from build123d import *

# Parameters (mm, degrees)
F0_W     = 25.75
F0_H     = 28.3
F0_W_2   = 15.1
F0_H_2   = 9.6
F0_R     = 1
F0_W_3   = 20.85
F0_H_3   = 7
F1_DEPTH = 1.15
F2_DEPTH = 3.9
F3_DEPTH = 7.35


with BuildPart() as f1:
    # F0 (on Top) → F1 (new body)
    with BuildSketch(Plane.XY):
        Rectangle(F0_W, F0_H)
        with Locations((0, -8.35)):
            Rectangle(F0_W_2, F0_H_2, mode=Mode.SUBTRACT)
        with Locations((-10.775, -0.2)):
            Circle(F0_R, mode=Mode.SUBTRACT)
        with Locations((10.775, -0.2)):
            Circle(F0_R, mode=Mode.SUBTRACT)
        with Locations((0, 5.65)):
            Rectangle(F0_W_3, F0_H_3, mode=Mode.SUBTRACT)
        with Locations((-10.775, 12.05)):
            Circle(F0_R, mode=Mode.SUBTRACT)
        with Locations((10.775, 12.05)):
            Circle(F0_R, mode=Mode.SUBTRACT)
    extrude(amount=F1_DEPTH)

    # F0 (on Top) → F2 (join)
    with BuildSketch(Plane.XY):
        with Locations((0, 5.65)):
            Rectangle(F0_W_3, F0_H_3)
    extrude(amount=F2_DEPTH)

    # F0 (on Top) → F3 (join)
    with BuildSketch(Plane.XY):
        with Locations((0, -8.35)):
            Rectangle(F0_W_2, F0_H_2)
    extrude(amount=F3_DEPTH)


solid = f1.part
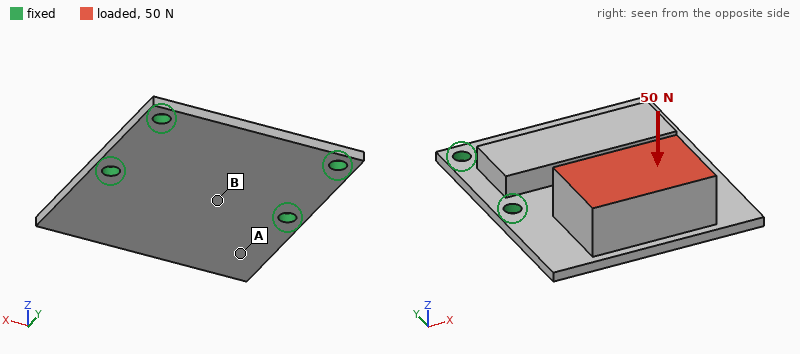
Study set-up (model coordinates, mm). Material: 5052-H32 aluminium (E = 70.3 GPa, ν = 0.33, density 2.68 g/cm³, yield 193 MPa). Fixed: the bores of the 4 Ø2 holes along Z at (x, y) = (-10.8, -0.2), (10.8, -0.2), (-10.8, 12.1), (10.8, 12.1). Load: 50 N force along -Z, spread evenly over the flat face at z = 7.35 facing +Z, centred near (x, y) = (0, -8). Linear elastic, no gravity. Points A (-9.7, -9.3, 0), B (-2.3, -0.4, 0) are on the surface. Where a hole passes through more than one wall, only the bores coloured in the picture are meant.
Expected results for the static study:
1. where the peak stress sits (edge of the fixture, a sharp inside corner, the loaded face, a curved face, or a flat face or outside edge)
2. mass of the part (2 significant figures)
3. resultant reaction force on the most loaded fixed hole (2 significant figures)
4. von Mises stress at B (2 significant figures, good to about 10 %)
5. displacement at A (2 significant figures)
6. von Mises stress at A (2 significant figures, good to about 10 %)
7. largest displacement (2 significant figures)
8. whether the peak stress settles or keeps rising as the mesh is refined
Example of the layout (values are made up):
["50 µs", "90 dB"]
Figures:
["edge of the fixture", "5.7 g", "32 N", "31 MPa", "44 µm", "11 MPa", "78 µm", "keeps rising"]
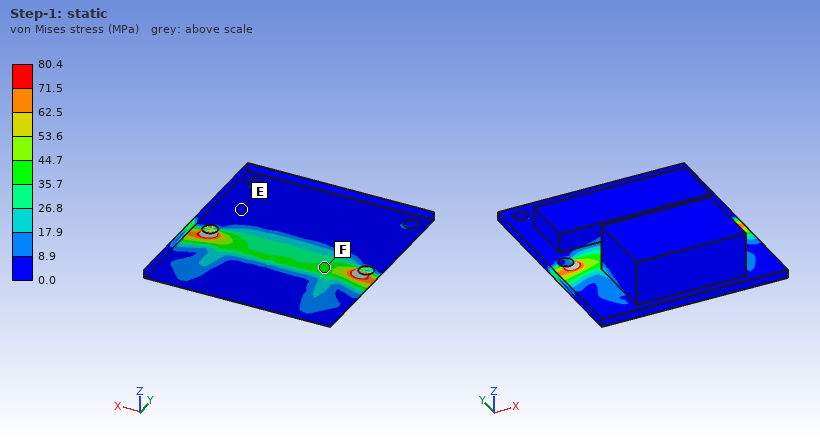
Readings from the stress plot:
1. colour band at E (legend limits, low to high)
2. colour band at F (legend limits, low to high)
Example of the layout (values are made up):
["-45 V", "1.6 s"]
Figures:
["0.0 to 8.9 MPa", "35.7 to 44.7 MPa"]
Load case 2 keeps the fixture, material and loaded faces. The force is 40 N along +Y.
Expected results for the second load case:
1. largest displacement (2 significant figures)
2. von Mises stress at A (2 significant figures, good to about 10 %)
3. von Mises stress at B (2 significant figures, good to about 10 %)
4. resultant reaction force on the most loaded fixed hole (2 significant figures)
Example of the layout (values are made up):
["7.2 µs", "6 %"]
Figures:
["64 µm", "6.9 MPa", "26 MPa", "14 N"]
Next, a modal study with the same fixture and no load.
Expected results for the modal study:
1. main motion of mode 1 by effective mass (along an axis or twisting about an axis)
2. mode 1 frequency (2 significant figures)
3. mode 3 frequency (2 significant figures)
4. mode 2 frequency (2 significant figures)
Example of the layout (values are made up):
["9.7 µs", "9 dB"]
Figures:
["along Z", "2600 Hz", "15 kHz", "11 kHz"]
